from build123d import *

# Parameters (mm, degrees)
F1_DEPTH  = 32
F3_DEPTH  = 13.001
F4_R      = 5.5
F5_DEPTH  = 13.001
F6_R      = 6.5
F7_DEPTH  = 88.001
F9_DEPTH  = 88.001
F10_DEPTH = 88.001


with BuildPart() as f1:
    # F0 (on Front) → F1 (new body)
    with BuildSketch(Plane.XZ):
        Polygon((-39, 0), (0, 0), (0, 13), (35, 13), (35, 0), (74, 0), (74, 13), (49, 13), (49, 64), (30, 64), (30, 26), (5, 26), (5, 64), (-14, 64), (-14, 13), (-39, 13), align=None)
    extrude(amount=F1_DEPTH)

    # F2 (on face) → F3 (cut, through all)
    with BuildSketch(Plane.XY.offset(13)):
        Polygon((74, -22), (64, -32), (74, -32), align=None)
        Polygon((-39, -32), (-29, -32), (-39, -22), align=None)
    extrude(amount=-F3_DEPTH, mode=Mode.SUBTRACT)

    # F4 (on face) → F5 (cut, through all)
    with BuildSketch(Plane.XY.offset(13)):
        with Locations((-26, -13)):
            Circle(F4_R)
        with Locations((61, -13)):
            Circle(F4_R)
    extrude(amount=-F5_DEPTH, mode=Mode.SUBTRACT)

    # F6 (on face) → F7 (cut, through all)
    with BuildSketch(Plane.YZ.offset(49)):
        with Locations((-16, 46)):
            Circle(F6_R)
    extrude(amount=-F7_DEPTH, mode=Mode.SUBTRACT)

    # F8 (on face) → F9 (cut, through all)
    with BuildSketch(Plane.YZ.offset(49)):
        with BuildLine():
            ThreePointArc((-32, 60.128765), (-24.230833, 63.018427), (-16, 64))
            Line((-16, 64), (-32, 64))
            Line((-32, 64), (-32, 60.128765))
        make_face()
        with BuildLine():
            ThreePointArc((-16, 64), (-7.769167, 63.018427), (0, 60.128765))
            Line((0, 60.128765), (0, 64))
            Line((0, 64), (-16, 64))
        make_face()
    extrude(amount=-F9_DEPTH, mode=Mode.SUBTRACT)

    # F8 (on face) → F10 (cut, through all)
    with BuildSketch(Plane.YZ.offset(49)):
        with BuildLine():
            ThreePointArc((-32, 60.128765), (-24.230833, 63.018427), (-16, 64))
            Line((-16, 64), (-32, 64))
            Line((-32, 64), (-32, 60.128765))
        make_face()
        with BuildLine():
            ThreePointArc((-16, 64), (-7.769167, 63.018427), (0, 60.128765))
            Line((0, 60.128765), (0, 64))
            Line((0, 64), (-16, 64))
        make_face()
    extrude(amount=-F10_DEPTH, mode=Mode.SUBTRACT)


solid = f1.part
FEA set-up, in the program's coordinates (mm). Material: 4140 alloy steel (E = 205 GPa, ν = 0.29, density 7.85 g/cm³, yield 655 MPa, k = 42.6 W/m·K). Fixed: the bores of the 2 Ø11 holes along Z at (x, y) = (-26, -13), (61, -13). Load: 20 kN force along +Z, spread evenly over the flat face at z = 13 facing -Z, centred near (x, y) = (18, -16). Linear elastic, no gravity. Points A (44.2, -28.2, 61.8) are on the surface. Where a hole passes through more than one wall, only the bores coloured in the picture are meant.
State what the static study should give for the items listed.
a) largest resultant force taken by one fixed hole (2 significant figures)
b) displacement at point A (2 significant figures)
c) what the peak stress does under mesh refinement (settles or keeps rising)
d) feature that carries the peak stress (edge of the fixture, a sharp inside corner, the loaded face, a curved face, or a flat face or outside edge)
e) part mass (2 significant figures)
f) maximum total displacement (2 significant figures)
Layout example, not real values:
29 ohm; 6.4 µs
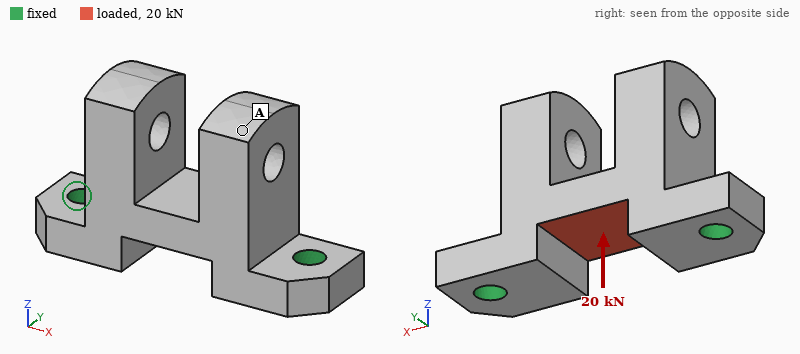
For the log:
15 kN; 35 µm; keeps rising; edge of the fixture; 740 g; 40 µm
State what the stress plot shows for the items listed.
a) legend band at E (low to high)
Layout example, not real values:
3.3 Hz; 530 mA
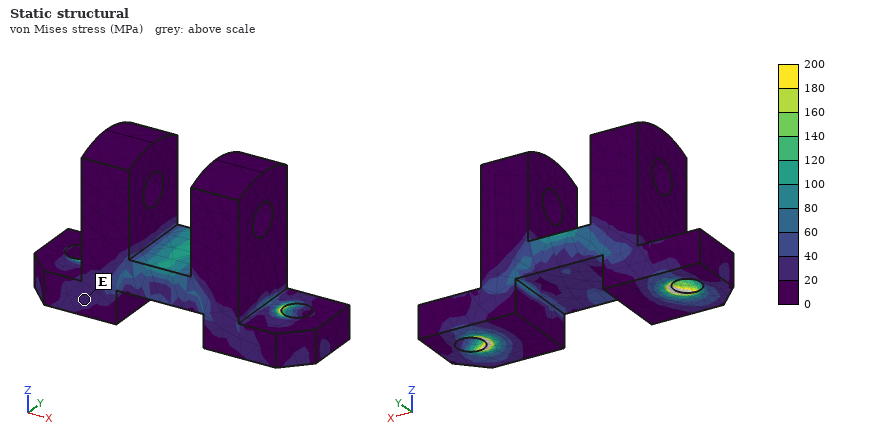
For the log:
20 to 40 MPa
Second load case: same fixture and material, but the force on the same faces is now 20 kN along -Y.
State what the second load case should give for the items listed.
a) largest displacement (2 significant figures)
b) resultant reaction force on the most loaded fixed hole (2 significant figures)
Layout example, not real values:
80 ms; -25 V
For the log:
48 µm; 10 kN
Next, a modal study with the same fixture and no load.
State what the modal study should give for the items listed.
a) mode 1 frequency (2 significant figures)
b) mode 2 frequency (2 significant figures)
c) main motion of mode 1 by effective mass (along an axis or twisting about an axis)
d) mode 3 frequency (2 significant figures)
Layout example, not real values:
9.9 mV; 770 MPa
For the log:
2900 Hz; 4500 Hz; along Y; 5100 Hz
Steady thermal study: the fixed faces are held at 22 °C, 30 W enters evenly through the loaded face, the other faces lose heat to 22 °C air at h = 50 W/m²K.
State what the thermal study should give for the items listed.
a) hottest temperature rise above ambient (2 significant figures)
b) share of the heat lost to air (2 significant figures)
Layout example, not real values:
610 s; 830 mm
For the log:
24 K; 33 %
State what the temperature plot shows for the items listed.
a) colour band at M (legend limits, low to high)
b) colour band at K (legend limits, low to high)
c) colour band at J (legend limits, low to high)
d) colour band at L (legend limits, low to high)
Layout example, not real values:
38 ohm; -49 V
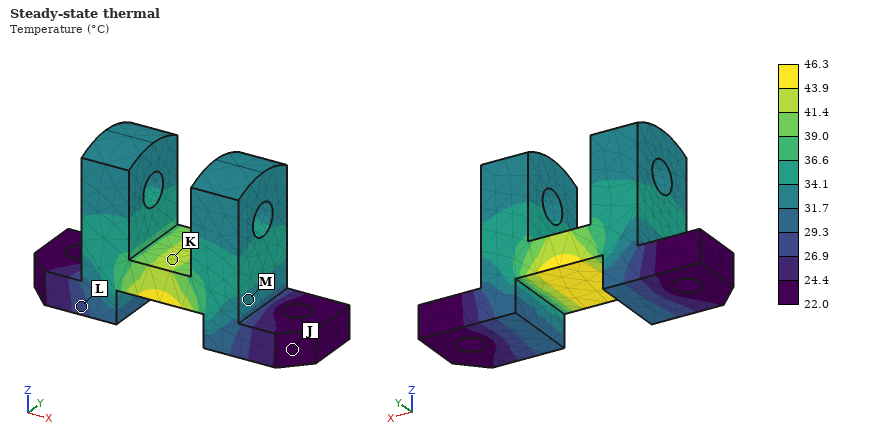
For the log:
31.7 to 34.1 °C; 41.4 to 43.9 °C; 22.0 to 24.4 °C; 26.9 to 29.3 °C
